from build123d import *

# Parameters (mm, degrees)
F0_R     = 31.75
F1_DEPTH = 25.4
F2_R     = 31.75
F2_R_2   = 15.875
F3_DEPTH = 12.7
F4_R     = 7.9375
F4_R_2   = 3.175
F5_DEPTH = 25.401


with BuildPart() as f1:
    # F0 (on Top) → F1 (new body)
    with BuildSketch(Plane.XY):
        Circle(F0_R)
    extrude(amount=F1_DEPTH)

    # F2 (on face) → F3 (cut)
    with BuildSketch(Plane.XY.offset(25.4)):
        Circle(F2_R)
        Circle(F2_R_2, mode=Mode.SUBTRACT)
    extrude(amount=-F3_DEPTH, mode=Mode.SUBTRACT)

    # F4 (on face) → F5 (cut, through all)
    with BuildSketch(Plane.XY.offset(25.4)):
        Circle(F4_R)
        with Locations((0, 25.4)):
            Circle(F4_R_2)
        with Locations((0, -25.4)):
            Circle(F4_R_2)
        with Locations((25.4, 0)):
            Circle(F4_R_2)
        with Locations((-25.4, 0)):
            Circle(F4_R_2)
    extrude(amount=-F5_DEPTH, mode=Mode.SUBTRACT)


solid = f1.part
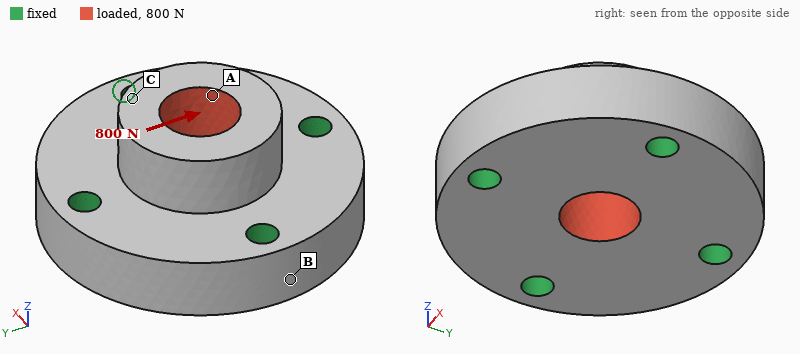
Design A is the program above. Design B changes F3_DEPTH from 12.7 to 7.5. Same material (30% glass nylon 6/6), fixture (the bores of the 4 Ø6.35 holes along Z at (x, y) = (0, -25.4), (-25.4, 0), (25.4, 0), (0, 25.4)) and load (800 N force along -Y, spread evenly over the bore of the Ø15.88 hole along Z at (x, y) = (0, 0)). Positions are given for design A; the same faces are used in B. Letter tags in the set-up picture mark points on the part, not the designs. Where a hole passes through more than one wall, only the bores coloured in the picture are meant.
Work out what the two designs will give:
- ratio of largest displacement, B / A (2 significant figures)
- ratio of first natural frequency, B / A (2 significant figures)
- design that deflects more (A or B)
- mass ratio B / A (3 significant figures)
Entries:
0.52
1.2
A
1.27
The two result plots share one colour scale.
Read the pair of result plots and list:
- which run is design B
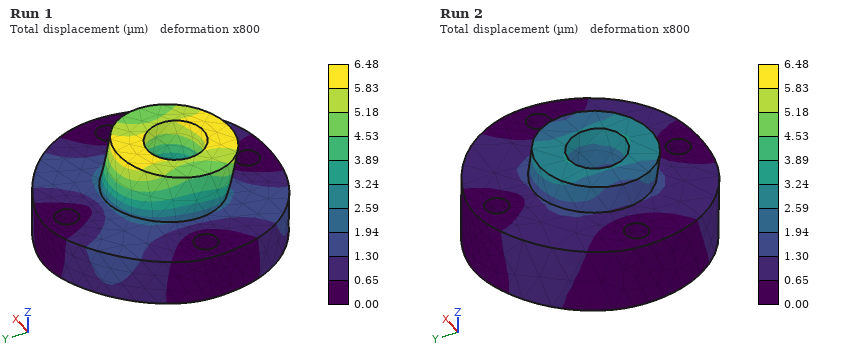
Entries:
Run 2
